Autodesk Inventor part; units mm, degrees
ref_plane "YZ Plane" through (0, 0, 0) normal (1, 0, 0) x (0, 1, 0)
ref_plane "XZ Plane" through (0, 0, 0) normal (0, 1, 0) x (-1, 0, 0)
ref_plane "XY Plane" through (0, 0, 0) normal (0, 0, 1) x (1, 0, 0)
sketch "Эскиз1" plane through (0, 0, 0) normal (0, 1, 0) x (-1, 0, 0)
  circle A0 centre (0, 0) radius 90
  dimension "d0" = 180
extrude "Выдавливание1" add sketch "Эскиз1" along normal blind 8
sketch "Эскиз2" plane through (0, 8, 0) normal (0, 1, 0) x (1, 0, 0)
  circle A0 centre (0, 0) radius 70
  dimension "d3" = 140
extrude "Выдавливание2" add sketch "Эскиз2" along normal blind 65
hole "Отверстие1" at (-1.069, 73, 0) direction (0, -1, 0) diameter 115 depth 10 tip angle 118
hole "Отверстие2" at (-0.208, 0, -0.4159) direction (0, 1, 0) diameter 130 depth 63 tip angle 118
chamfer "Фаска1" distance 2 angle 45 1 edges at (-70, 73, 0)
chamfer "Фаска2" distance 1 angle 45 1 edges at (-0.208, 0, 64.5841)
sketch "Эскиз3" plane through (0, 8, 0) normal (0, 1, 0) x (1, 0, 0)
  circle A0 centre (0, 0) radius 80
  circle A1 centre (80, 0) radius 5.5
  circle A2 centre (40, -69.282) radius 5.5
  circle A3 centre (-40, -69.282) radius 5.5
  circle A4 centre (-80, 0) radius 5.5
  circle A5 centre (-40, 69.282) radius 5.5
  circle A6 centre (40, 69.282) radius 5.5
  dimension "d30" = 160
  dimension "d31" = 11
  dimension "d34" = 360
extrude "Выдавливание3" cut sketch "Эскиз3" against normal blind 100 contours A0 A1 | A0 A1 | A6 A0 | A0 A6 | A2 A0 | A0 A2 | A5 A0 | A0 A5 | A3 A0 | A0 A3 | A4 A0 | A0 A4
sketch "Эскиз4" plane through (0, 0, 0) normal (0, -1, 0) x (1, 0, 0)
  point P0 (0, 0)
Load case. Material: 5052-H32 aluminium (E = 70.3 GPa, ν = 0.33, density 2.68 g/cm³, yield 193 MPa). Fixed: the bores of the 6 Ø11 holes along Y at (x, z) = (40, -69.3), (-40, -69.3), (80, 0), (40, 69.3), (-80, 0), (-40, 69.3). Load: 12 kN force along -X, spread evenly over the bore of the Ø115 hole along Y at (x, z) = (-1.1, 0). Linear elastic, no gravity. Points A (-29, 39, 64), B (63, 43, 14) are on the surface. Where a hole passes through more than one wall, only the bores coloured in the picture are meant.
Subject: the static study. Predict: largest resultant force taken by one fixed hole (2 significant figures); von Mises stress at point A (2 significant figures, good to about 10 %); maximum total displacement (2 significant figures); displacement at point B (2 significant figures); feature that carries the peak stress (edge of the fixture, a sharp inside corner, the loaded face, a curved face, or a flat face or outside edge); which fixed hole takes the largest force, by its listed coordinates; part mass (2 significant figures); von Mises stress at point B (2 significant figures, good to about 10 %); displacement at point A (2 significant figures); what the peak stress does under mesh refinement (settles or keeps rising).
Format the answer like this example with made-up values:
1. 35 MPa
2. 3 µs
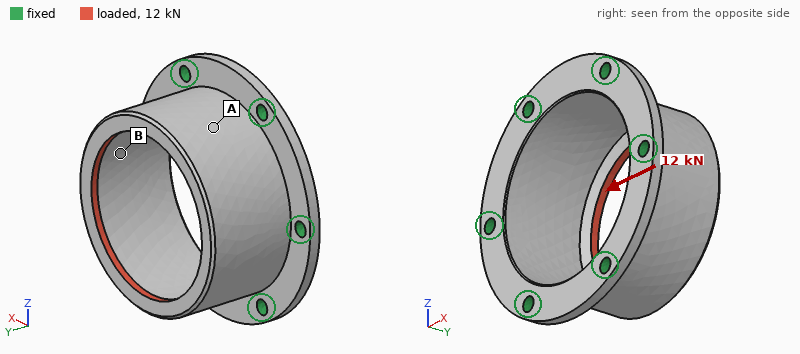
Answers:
1. 4.2 kN
2. 16 MPa
3. 88 µm
4. 26 µm
5. edge of the fixture
6. (-80, 0)
7. 680 g
8. 7.2 MPa
9. 25 µm
10. keeps rising
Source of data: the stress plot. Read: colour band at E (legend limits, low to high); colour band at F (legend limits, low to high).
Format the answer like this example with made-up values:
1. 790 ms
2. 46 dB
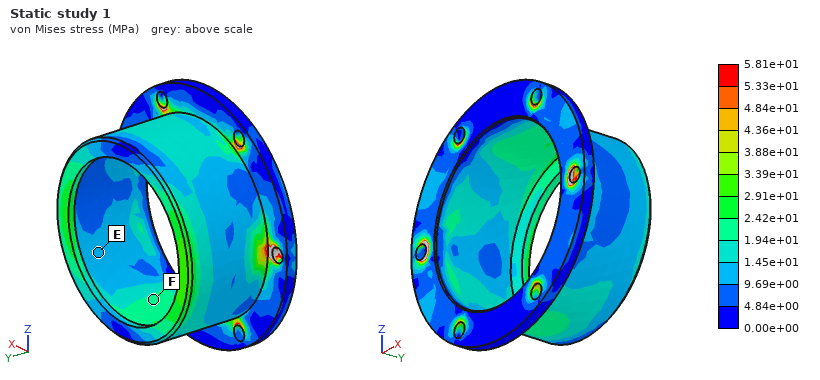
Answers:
1. 9.69e+00 to 1.45e+01 MPa
2. 1.94e+01 to 2.42e+01 MPa
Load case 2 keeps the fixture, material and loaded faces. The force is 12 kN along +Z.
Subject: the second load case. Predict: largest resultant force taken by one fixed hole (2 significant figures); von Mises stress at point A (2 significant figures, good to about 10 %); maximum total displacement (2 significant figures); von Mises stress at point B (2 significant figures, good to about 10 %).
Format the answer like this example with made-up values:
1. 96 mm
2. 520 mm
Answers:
1. 4.0 kN
2. 11 MPa
3. 79 µm
4. 18 MPa
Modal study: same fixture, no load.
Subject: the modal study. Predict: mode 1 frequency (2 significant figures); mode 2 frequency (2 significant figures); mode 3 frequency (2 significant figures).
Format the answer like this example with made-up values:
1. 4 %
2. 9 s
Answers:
1. 3000 Hz
2. 3000 Hz
3. 4500 Hz
